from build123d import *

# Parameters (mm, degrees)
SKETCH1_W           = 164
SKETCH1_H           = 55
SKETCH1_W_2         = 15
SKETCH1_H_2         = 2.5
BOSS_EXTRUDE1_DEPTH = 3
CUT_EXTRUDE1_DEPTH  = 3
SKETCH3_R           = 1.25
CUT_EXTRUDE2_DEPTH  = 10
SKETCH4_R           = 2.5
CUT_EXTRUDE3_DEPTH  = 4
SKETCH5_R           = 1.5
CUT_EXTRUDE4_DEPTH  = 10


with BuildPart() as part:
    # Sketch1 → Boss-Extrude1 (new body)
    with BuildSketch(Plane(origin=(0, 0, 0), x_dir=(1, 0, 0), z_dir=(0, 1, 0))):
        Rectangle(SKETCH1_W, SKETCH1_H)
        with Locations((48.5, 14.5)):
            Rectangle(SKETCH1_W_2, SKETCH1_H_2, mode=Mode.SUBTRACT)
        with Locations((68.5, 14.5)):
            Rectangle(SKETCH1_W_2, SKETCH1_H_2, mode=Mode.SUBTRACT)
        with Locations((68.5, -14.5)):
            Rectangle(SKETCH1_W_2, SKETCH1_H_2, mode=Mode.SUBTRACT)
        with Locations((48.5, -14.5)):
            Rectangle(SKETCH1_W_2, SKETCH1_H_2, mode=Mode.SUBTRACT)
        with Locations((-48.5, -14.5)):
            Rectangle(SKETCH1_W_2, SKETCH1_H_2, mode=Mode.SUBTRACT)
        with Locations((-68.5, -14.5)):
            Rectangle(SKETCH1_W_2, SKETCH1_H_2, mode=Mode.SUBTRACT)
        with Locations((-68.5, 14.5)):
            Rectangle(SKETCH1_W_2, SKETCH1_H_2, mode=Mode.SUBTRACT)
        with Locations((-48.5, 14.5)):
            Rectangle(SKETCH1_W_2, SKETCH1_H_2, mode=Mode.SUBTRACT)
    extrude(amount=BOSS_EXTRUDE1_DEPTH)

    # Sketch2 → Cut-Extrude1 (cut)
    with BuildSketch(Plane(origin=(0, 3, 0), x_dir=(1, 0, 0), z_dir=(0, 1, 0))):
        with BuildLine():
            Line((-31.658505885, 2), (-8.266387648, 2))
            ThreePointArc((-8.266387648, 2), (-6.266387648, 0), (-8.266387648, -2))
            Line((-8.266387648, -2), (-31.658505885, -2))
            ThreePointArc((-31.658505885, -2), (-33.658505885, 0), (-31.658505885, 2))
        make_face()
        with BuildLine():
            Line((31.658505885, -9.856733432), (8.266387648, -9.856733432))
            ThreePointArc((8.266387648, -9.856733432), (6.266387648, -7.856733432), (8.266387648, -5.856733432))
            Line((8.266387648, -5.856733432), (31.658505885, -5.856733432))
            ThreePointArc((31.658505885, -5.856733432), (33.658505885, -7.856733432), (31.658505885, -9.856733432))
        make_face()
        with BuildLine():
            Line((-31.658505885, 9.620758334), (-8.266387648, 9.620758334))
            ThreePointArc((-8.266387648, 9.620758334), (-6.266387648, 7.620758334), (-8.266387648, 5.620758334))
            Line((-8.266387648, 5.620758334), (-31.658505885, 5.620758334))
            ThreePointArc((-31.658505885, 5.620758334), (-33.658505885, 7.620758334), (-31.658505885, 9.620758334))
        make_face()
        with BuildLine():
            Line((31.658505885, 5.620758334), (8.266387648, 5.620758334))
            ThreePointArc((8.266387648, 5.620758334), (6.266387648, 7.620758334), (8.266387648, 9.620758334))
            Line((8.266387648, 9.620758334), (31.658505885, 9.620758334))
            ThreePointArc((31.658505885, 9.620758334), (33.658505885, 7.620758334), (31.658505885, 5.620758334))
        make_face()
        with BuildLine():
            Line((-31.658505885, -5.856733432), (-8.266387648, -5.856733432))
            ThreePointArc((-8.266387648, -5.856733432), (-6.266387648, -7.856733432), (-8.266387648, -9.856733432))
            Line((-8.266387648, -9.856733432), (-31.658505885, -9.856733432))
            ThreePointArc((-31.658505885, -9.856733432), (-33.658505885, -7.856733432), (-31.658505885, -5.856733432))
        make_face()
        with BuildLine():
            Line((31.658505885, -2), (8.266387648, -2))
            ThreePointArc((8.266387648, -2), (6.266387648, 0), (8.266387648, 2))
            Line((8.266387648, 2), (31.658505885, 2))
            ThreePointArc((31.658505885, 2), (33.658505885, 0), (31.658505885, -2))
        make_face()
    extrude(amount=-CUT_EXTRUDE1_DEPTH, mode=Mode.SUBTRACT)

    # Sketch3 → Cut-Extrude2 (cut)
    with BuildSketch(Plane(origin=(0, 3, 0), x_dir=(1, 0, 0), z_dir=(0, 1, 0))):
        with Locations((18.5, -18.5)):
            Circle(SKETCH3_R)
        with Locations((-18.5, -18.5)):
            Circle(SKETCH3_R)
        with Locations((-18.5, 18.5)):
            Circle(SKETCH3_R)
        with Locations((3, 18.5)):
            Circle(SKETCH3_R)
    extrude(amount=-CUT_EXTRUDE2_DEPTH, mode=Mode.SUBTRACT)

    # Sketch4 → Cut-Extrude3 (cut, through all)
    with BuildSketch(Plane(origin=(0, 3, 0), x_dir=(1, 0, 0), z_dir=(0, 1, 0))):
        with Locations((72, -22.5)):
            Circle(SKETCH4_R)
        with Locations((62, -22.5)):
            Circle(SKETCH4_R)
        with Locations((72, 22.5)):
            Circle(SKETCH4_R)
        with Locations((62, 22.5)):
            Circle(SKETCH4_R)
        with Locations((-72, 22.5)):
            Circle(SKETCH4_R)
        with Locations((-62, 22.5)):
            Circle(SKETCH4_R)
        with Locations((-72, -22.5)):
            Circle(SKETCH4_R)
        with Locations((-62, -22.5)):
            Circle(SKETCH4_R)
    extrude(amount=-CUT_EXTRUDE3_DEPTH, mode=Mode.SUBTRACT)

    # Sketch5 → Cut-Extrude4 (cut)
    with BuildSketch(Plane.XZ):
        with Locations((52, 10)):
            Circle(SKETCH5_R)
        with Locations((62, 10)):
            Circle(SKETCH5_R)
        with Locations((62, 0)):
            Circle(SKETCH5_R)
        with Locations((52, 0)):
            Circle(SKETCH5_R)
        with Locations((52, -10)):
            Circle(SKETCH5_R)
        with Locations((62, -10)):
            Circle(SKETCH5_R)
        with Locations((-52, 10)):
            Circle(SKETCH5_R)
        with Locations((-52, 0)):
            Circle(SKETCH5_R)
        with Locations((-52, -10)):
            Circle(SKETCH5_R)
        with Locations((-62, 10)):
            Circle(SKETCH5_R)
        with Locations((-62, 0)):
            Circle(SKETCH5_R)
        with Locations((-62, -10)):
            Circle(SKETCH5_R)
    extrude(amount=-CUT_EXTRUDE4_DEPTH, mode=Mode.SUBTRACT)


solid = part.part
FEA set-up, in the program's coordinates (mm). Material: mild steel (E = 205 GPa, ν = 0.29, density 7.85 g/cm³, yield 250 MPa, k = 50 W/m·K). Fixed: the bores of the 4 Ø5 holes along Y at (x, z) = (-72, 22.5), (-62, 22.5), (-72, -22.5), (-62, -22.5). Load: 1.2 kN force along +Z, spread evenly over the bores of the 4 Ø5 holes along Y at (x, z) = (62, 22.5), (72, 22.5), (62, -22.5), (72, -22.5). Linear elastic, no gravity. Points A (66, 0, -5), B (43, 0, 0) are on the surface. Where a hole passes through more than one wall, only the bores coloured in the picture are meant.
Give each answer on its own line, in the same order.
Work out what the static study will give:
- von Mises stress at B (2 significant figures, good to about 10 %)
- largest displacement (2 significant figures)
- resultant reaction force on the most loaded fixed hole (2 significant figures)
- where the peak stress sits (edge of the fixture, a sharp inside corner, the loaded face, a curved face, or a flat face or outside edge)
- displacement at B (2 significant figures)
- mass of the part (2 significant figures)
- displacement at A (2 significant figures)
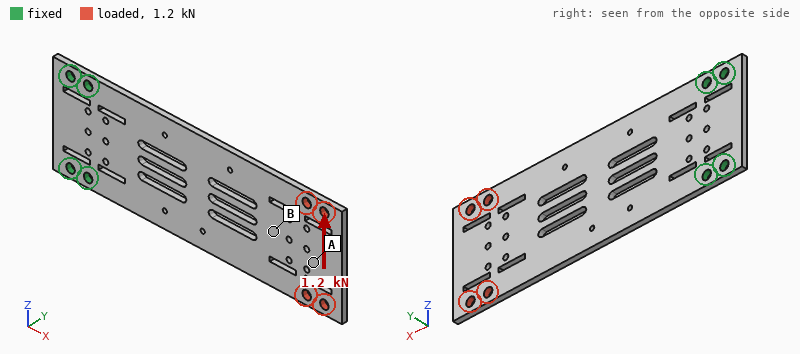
33 MPa
0.18 mm
3.1 kN
a curved face
0.12 mm
180 g
0.16 mm
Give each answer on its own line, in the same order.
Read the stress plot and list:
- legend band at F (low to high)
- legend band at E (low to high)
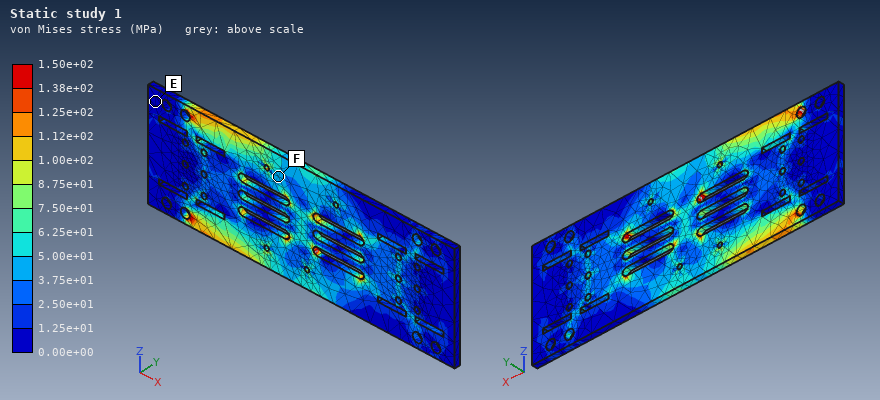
3.75e+01 to 5.00e+01 MPa
0.00e+00 to 1.25e+01 MPa
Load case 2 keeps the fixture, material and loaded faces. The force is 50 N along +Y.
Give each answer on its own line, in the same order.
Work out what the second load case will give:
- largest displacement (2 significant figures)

2.0 mm
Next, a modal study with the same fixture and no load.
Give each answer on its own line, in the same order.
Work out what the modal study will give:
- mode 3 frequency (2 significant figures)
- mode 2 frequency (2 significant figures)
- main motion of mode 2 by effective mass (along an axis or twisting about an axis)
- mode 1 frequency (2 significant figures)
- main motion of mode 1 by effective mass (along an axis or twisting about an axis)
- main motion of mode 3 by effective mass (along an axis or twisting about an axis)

730 Hz
610 Hz
twisting about X
120 Hz
along Y
along Y
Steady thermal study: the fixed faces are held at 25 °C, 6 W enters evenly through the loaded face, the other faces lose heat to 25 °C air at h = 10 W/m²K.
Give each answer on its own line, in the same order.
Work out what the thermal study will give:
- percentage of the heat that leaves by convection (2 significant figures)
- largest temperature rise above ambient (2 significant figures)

72 %
59 K
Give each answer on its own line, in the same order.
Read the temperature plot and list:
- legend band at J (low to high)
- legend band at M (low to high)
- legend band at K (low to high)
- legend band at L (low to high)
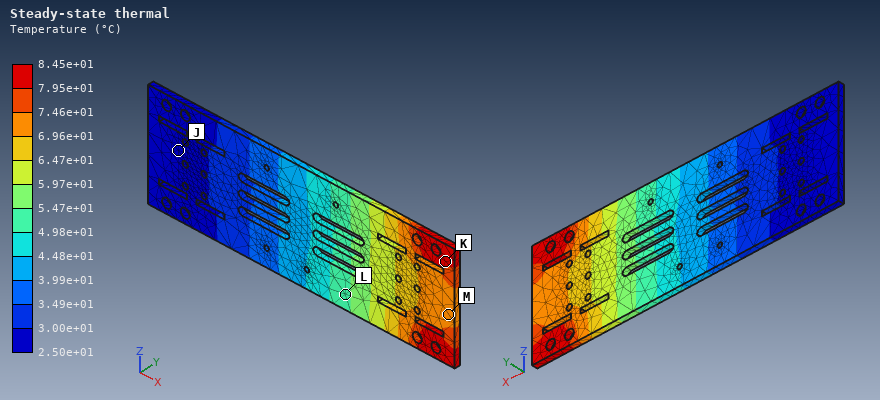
2.50e+01 to 3.00e+01 °C
6.96e+01 to 7.46e+01 °C
7.95e+01 to 8.45e+01 °C
4.98e+01 to 5.47e+01 °C
